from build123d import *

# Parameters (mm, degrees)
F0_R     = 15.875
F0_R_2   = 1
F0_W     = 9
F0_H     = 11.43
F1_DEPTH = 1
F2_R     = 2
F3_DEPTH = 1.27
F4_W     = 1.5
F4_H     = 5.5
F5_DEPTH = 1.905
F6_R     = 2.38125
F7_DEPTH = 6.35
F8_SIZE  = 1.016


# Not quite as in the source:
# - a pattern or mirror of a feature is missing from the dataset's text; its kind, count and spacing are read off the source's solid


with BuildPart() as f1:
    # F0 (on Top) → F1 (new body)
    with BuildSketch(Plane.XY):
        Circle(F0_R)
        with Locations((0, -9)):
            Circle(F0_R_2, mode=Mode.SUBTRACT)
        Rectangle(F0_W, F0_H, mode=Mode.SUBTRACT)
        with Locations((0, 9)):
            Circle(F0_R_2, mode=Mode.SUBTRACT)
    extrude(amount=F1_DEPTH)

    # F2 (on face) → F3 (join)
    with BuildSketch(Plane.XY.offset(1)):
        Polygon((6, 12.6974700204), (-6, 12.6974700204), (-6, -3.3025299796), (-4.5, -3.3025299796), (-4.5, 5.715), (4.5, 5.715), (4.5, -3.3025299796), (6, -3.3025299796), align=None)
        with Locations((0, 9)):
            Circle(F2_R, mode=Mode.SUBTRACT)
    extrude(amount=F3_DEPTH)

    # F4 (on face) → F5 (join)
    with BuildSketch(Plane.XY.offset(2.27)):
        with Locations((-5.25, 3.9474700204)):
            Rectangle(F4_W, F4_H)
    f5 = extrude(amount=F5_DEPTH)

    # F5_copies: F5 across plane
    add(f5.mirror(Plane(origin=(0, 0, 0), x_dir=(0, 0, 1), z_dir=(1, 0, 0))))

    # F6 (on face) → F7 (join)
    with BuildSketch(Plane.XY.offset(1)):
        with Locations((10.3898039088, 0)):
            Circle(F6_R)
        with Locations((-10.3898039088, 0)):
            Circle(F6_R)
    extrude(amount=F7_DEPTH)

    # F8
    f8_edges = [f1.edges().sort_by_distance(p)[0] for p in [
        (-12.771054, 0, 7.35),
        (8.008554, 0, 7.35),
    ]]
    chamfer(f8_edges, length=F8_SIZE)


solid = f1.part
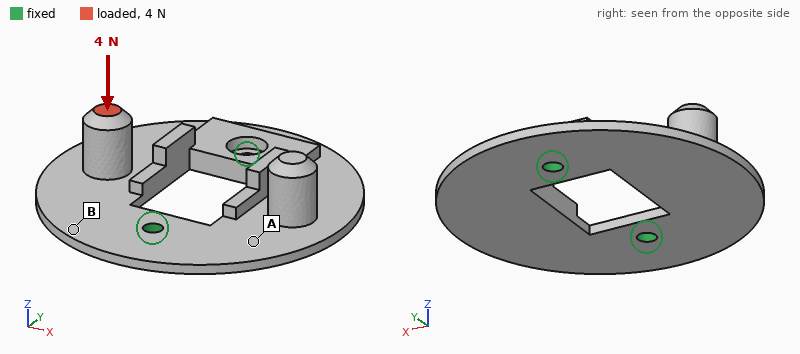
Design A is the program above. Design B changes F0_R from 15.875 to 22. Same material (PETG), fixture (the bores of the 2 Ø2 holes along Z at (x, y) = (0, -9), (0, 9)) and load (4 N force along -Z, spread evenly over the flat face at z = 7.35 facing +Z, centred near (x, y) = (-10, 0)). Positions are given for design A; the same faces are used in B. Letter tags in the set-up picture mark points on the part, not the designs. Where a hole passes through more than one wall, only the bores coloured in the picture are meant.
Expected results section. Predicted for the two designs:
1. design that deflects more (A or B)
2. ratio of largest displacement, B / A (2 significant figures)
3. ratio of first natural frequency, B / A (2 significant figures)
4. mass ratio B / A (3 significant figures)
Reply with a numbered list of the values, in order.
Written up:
1. B
2. 1.2
3. 0.60
4. 1.69
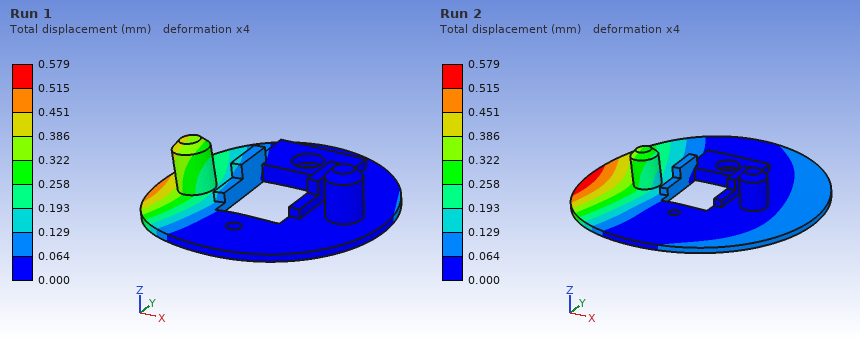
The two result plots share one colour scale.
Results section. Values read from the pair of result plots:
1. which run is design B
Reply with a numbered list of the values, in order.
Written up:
1. Run 2
